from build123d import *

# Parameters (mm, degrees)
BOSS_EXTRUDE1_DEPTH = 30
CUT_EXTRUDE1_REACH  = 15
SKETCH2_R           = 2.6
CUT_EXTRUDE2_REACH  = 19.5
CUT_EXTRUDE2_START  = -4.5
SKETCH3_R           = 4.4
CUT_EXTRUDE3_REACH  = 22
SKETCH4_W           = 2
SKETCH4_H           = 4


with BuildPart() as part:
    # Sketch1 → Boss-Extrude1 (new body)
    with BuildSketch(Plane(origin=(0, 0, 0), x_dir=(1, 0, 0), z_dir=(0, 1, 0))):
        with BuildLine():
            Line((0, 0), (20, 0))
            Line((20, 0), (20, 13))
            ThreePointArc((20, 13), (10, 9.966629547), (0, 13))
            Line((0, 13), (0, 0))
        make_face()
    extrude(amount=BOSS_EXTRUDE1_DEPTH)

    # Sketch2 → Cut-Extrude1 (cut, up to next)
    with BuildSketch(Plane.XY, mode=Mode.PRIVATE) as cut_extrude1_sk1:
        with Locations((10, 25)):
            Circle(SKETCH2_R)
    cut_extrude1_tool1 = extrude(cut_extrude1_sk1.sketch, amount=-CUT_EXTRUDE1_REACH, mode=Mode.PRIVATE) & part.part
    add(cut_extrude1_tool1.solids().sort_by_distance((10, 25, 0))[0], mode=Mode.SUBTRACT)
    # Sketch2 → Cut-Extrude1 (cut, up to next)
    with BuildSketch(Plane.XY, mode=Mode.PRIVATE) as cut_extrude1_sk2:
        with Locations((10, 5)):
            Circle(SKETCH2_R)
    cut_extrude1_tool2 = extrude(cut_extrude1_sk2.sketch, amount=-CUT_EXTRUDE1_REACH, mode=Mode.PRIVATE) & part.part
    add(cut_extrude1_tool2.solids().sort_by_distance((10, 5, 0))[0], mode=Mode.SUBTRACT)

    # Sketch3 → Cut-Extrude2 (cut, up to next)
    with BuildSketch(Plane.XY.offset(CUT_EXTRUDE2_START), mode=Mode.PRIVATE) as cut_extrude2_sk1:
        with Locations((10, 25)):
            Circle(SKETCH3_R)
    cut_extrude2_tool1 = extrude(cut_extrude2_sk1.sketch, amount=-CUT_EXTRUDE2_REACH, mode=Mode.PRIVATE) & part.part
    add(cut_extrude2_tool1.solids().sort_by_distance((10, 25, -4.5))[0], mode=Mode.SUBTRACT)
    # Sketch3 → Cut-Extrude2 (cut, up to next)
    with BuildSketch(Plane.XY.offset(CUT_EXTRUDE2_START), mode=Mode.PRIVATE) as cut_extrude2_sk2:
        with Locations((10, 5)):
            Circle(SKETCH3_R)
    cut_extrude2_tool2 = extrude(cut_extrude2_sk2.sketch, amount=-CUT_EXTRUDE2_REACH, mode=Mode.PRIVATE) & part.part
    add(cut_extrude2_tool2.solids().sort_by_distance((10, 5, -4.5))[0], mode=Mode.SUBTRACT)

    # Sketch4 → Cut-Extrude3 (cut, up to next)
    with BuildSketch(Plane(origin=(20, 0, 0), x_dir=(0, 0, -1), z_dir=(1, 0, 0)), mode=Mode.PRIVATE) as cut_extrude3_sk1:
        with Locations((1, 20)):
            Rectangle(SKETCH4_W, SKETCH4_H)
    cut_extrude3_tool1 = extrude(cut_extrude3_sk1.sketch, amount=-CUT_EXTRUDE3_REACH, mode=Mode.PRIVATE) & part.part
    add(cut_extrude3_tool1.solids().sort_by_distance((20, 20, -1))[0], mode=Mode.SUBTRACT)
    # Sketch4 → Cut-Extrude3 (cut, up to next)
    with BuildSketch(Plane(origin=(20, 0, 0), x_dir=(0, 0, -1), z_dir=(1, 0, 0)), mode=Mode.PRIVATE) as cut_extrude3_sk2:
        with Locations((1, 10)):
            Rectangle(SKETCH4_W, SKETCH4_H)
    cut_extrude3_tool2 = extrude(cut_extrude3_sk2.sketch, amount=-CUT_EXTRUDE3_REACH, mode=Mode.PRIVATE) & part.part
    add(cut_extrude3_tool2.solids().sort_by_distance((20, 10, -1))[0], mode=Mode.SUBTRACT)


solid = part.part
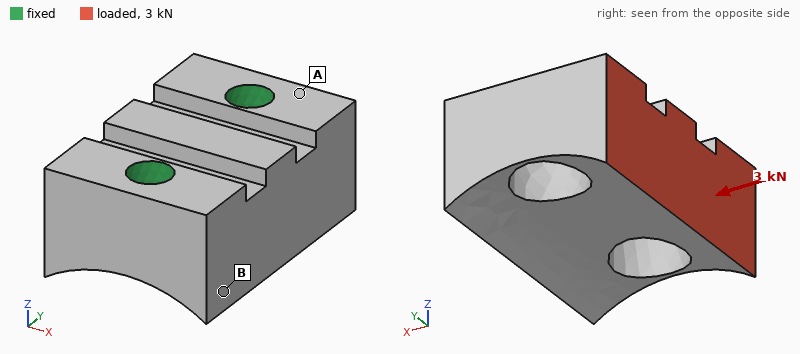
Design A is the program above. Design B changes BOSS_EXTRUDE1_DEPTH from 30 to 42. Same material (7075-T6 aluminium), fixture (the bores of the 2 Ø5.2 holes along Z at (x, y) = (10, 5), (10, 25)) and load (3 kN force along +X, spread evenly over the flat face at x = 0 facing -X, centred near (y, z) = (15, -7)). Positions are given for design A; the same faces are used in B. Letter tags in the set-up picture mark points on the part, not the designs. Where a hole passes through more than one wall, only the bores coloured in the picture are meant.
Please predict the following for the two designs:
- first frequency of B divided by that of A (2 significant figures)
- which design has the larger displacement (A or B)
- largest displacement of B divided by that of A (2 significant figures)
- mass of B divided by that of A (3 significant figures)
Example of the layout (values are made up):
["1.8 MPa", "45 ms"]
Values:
["0.78", "B", "1.2", "1.49"]
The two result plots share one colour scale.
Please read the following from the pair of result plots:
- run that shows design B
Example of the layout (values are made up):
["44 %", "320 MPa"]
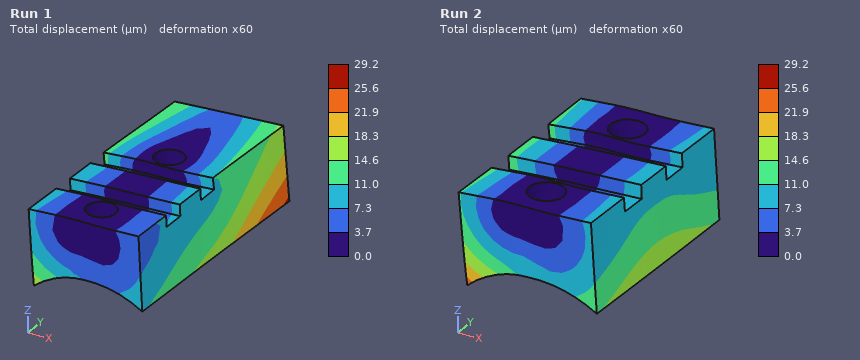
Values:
["Run 1"]
